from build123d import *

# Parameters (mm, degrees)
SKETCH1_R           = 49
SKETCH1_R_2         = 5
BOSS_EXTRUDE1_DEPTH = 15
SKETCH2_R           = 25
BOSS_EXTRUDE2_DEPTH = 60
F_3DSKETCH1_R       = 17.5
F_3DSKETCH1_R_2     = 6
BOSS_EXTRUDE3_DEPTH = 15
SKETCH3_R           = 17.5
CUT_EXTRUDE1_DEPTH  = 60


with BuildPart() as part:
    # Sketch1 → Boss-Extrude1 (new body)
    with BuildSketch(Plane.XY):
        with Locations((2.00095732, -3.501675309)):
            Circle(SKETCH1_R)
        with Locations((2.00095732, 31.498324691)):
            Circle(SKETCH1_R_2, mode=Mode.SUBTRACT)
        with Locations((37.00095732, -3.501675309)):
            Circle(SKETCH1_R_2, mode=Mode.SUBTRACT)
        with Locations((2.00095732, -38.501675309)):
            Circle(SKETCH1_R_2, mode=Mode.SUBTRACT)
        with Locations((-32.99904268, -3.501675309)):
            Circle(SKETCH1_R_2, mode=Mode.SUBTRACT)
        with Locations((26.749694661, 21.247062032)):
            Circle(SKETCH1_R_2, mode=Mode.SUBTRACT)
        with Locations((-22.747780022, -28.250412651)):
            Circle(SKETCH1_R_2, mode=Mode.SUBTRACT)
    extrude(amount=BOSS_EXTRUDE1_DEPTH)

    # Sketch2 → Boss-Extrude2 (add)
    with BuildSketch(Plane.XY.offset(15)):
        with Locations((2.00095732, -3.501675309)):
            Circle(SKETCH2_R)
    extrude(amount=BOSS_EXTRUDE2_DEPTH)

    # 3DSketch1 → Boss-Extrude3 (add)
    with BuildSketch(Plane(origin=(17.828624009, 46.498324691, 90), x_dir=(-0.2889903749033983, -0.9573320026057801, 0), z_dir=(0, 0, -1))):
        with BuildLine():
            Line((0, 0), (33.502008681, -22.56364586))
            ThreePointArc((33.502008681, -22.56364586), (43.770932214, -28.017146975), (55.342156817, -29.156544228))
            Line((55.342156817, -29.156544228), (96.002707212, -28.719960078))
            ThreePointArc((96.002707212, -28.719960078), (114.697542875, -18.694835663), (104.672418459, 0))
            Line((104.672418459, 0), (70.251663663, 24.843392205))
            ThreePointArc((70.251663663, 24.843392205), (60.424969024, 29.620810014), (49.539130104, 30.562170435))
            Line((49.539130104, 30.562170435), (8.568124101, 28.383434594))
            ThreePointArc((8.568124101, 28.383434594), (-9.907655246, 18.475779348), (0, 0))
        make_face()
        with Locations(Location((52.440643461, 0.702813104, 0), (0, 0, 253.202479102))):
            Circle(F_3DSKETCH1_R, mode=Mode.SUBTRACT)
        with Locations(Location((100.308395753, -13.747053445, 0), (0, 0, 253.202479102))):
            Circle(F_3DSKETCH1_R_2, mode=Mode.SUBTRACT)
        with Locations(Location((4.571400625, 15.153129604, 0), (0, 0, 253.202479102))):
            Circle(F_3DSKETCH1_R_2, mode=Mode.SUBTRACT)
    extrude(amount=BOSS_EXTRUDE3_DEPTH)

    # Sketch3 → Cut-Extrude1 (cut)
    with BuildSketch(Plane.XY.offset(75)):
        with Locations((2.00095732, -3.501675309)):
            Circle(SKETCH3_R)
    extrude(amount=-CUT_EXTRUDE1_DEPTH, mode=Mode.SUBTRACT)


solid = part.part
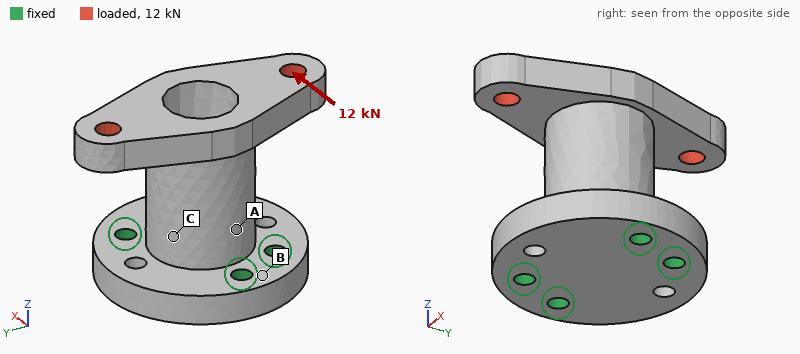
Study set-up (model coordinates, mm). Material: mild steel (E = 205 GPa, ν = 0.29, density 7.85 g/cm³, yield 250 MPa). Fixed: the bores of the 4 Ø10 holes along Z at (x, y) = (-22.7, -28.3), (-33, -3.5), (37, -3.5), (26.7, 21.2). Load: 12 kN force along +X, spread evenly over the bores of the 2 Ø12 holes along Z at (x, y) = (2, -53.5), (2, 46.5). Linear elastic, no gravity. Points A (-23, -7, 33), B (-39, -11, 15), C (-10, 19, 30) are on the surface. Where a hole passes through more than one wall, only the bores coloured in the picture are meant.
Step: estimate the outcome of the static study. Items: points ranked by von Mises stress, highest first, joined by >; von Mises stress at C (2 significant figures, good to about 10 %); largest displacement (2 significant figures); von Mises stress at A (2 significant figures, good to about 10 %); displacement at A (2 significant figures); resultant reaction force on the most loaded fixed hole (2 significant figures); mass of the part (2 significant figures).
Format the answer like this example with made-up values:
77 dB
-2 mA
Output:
A > C > B
37 MPa
83 µm
60 MPa
19 µm
13 kN
1.8 kg
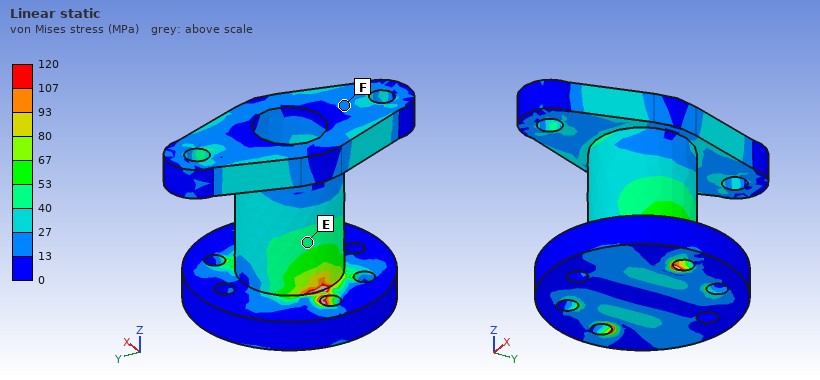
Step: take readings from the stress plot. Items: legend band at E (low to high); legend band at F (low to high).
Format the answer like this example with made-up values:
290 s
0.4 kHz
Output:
40 to 53 MPa
13 to 27 MPa
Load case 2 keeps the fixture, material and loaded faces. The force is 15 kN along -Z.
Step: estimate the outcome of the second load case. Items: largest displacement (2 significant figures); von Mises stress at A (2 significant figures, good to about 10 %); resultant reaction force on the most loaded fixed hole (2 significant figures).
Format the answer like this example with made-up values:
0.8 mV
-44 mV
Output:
0.13 mm
17 MPa
4.3 kN
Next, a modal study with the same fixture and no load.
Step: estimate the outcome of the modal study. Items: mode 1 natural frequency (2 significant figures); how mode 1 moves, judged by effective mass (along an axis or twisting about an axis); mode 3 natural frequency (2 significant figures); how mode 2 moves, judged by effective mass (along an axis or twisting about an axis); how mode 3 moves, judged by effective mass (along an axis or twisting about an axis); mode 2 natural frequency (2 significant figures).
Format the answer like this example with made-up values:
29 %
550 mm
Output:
2100 Hz
along Y
4100 Hz
along X
twisting about Z
2800 Hz
